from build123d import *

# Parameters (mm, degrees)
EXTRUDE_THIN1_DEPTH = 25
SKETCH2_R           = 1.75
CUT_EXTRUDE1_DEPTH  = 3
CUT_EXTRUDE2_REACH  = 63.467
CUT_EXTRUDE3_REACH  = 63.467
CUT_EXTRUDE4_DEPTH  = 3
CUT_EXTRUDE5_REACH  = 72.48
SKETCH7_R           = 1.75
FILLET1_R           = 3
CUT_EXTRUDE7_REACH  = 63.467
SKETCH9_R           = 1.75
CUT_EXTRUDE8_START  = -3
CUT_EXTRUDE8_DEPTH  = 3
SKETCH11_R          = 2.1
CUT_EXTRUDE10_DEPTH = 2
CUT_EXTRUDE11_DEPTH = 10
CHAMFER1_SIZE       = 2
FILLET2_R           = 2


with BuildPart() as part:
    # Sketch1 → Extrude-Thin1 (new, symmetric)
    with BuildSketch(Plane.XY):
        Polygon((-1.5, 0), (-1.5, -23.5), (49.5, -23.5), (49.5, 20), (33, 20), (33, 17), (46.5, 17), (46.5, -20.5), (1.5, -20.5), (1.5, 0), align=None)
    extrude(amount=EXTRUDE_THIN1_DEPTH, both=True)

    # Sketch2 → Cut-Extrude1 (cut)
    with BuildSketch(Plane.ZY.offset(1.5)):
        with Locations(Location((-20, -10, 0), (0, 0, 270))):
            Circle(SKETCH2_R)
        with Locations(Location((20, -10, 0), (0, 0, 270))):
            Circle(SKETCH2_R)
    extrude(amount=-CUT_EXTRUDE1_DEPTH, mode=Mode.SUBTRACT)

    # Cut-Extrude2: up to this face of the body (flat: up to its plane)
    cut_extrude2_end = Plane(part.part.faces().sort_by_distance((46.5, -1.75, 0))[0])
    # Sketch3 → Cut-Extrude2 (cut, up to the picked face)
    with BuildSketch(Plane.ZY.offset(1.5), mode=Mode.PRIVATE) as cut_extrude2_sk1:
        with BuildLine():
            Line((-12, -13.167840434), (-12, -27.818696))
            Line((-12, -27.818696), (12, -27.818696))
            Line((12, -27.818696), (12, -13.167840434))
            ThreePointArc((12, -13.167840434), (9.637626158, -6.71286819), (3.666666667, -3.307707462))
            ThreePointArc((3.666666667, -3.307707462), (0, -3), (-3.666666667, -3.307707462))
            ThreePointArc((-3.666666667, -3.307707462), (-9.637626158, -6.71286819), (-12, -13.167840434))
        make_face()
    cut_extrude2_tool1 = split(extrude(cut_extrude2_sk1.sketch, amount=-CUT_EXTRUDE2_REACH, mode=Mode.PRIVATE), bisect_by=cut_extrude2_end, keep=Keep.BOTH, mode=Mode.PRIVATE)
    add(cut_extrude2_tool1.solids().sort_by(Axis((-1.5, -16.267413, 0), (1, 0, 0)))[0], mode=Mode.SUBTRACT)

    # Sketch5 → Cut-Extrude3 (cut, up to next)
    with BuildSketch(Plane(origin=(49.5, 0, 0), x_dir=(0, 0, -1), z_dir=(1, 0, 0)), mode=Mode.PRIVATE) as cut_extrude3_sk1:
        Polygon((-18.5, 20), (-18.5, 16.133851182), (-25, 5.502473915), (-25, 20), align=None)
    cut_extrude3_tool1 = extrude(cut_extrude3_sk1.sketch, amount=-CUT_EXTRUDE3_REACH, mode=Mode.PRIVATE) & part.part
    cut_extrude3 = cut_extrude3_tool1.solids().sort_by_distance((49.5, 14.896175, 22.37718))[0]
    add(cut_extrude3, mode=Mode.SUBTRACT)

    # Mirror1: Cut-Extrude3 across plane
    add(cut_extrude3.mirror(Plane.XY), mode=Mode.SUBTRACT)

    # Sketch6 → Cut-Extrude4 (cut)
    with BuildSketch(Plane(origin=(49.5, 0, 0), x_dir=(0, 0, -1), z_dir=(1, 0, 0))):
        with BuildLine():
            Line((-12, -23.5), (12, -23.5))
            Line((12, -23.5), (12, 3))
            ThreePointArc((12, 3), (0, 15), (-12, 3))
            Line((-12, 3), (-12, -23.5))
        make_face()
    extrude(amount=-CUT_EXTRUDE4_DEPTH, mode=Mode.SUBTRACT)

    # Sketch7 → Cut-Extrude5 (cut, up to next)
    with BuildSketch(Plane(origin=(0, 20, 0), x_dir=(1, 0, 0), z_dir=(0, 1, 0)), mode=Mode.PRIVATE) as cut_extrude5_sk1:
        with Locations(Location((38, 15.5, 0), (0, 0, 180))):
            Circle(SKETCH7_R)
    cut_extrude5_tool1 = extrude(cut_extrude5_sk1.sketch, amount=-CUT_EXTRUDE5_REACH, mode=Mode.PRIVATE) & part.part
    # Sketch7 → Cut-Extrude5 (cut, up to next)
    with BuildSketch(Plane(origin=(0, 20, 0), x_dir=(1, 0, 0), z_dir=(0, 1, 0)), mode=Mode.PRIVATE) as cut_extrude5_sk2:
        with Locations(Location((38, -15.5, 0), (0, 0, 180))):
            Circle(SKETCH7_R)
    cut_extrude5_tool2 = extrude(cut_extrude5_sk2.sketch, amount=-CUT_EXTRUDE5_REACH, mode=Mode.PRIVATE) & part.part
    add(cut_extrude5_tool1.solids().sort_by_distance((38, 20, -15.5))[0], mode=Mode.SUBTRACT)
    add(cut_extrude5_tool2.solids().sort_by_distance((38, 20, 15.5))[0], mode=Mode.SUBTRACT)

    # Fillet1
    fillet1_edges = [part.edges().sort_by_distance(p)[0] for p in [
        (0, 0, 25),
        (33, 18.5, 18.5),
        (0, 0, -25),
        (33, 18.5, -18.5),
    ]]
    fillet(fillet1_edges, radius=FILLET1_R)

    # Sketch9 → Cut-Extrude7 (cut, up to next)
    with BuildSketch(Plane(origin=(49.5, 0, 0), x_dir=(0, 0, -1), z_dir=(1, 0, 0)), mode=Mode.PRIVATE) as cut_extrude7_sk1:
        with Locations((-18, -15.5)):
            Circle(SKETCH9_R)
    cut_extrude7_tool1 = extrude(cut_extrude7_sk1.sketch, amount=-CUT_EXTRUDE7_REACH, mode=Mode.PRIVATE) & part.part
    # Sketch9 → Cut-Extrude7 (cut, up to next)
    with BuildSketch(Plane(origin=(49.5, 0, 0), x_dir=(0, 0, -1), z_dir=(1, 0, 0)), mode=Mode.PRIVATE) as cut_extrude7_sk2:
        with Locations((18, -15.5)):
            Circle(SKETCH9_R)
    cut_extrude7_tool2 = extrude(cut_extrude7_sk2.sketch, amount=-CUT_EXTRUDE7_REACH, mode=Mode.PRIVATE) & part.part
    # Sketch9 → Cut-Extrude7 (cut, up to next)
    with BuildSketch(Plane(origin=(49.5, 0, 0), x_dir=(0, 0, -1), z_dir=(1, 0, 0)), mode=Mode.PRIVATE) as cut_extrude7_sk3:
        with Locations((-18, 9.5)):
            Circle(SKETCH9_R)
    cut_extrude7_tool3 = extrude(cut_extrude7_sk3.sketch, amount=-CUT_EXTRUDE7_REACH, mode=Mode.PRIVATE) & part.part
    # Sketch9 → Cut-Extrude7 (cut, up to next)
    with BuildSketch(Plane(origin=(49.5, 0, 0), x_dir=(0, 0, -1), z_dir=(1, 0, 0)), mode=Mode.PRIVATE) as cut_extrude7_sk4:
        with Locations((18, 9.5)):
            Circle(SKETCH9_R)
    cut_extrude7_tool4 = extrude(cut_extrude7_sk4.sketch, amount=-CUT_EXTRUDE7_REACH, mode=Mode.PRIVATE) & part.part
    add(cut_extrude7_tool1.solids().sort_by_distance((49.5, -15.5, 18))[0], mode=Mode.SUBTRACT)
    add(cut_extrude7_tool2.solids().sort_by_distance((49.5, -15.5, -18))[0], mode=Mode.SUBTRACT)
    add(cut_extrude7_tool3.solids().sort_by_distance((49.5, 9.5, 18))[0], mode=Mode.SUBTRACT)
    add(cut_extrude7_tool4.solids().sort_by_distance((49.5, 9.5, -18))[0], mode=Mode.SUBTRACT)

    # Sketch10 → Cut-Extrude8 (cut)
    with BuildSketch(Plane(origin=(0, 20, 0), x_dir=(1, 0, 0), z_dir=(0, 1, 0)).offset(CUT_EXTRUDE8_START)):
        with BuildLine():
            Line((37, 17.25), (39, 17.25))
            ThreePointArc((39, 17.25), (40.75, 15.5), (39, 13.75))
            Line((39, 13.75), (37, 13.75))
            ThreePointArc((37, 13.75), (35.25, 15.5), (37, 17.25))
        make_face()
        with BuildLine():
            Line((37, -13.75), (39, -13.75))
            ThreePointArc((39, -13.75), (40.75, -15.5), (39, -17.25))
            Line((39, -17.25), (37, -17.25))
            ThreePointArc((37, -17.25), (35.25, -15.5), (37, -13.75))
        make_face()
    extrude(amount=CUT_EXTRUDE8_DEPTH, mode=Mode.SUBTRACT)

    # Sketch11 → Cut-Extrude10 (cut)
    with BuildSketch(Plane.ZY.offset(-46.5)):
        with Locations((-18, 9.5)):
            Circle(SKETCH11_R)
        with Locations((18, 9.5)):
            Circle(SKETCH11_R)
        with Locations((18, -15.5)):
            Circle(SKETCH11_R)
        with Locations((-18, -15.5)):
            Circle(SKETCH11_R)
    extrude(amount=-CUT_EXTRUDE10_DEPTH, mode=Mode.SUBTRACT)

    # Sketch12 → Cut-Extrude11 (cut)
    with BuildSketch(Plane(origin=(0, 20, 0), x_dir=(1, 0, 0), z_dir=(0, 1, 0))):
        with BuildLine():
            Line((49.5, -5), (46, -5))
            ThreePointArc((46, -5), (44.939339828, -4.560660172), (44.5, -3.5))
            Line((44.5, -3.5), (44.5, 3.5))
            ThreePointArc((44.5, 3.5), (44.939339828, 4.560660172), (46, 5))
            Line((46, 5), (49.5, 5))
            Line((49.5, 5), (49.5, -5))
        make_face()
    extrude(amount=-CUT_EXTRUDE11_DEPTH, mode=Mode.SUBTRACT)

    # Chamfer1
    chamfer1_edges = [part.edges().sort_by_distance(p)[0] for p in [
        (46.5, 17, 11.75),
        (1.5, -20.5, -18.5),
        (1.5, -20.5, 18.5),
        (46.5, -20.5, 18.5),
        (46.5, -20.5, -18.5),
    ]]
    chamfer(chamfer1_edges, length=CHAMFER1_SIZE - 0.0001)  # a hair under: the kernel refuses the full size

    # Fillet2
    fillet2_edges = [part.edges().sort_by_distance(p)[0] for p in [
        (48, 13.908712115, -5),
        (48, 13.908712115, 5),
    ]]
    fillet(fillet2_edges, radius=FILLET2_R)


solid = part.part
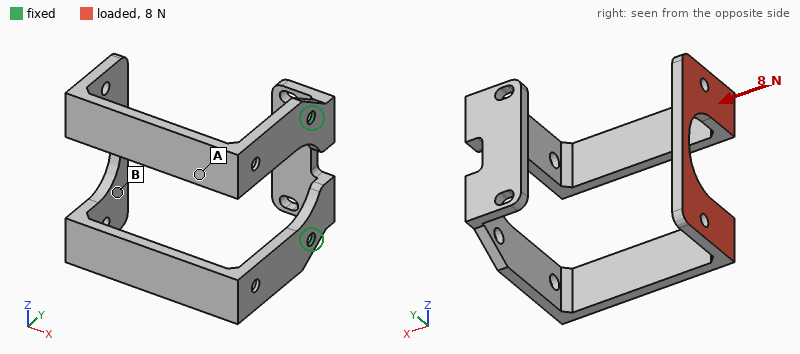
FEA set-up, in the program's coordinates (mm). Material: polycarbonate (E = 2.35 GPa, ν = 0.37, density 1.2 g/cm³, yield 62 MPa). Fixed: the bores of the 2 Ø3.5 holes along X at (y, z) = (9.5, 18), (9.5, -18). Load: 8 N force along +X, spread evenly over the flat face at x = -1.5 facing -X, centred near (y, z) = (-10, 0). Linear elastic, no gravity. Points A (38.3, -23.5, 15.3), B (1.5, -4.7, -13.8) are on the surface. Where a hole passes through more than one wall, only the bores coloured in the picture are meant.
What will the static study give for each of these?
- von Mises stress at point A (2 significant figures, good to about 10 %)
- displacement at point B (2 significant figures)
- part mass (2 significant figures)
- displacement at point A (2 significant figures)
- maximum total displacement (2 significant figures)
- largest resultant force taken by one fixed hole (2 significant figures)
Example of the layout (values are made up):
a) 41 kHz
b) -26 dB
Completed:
a) 2.2 MPa
b) 0.75 mm
c) 12 g
d) 0.45 mm
e) 0.86 mm
f) 4.0 N
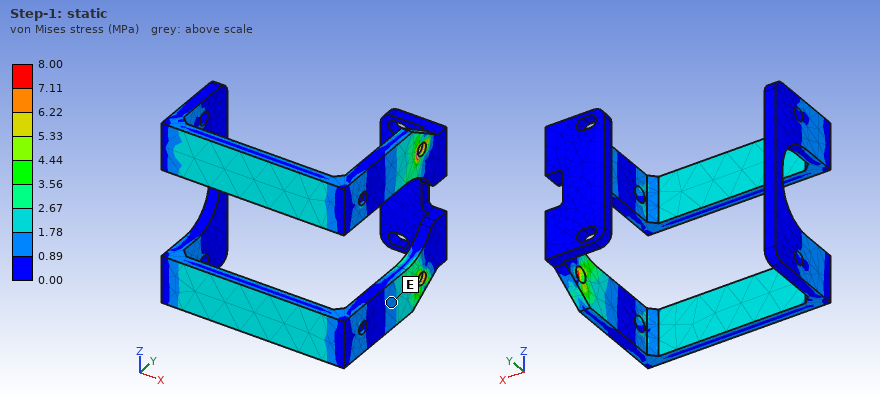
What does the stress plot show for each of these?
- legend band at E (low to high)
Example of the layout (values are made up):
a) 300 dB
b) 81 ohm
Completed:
a) 0.89 to 1.78 MPa
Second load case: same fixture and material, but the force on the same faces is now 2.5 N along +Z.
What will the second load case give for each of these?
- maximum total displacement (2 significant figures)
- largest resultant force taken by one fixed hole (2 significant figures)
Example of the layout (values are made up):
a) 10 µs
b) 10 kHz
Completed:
a) 1.0 mm
b) 2.5 N
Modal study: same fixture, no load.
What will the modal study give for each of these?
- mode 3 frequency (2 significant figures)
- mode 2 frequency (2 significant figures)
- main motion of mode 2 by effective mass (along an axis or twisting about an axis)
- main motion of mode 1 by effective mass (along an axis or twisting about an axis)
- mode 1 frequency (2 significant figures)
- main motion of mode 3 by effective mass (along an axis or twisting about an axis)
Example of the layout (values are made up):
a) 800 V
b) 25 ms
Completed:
a) 250 Hz
b) 130 Hz
c) along Z
d) along Y
e) 84 Hz
f) along X
